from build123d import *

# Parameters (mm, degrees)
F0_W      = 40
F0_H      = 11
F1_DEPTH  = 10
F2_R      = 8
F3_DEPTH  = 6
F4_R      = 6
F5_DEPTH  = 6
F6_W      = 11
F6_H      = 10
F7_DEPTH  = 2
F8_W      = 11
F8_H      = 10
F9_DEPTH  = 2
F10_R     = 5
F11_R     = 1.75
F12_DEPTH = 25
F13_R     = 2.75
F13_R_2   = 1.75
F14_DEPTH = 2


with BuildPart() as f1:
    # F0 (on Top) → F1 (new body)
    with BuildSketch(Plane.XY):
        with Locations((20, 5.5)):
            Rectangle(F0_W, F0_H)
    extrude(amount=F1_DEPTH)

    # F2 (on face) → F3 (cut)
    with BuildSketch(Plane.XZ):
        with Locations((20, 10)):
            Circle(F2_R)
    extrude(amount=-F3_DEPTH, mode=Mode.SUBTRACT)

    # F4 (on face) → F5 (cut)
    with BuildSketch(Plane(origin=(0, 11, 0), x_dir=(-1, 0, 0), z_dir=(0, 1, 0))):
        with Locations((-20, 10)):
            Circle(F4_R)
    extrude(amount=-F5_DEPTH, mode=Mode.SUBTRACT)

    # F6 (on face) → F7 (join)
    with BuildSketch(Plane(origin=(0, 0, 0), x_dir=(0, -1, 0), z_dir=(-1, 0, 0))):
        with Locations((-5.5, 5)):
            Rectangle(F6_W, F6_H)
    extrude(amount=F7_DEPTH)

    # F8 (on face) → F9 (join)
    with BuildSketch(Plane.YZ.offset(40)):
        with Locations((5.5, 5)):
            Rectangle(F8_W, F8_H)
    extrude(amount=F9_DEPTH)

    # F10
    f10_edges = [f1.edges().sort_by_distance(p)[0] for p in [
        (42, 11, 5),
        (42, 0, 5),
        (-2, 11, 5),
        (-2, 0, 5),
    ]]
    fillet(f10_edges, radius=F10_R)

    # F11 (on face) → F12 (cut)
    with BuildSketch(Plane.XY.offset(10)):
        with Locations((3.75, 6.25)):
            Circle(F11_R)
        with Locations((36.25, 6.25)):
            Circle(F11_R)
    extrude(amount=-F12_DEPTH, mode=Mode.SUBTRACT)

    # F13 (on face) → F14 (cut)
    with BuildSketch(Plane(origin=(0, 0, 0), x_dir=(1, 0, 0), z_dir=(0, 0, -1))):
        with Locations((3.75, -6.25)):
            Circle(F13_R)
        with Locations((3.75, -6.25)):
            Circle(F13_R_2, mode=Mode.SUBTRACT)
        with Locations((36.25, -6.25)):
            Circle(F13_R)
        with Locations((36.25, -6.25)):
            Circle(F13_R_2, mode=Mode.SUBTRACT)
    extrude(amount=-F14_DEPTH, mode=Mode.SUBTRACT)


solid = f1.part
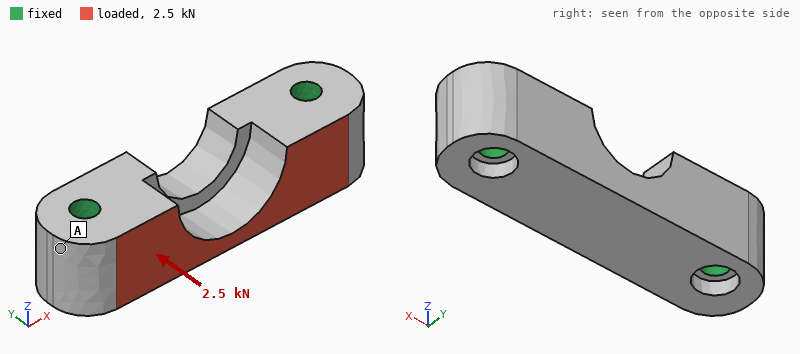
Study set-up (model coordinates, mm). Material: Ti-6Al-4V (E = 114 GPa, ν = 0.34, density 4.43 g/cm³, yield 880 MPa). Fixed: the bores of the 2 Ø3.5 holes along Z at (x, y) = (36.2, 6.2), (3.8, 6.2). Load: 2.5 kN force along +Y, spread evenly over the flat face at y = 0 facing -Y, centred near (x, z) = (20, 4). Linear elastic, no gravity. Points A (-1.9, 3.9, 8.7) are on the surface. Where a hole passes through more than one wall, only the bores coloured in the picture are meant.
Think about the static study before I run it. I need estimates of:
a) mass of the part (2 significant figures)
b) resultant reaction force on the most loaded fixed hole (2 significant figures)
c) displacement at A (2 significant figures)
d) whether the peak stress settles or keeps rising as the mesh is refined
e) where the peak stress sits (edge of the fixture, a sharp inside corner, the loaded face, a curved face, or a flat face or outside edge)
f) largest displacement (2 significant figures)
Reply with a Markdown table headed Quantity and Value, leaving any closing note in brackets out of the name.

| Quantity | Value |
|---|---|
| mass of the part | 15 g |
| resultant reaction force on the most loaded fixed hole | 1.3 kN |
| displacement at A | 1.5 µm |
| whether the peak stress settles or keeps rising as the mesh is refined | keeps rising |
| where the peak stress sits | edge of the fixture |
| largest displacement | 8.8 µm |
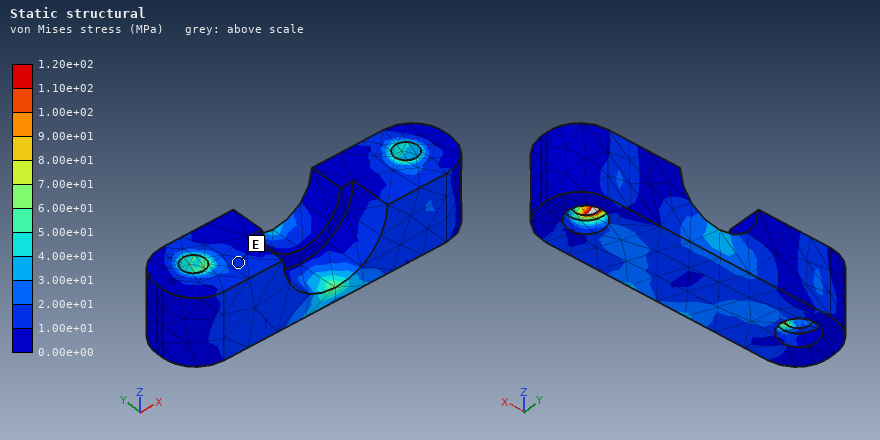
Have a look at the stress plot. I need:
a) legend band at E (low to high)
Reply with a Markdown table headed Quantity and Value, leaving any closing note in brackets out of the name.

| Quantity | Value |
|---|---|
| legend band at E | 1.00e+01 to 2.00e+01 MPa |
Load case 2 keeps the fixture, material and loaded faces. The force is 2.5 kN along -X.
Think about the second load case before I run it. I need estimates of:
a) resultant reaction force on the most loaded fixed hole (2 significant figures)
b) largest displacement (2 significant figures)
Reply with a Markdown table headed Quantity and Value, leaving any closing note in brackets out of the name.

| Quantity | Value |
|---|---|
| resultant reaction force on the most loaded fixed hole | 1.3 kN |
| largest displacement | 3.7 µm |
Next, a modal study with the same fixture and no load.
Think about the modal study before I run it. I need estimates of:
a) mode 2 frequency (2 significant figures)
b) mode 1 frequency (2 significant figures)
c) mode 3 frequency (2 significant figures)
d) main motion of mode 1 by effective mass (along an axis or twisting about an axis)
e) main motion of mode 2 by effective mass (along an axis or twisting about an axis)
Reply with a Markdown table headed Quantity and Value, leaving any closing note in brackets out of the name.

| Quantity | Value |
|---|---|
| mode 2 frequency | 37 kHz |
| mode 1 frequency | 30 kHz |
| mode 3 frequency | 51 kHz |
| main motion of mode 1 by effective mass | along Y |
| main motion of mode 2 by effective mass | along Z |
